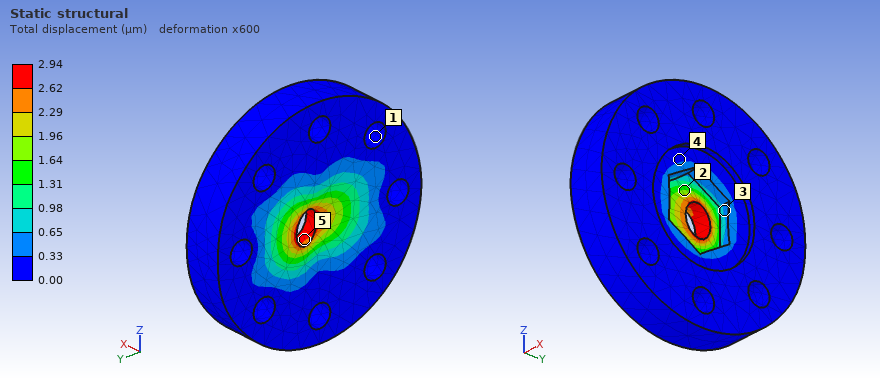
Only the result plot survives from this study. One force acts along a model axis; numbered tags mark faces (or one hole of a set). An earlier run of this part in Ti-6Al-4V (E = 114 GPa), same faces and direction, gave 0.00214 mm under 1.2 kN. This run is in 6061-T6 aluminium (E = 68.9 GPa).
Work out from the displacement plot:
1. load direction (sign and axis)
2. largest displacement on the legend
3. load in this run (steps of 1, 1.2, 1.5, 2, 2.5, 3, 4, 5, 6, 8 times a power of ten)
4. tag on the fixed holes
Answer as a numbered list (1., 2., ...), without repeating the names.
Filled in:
1. +Y
2. 2.94 µm
3. 1 kN
4. 1
